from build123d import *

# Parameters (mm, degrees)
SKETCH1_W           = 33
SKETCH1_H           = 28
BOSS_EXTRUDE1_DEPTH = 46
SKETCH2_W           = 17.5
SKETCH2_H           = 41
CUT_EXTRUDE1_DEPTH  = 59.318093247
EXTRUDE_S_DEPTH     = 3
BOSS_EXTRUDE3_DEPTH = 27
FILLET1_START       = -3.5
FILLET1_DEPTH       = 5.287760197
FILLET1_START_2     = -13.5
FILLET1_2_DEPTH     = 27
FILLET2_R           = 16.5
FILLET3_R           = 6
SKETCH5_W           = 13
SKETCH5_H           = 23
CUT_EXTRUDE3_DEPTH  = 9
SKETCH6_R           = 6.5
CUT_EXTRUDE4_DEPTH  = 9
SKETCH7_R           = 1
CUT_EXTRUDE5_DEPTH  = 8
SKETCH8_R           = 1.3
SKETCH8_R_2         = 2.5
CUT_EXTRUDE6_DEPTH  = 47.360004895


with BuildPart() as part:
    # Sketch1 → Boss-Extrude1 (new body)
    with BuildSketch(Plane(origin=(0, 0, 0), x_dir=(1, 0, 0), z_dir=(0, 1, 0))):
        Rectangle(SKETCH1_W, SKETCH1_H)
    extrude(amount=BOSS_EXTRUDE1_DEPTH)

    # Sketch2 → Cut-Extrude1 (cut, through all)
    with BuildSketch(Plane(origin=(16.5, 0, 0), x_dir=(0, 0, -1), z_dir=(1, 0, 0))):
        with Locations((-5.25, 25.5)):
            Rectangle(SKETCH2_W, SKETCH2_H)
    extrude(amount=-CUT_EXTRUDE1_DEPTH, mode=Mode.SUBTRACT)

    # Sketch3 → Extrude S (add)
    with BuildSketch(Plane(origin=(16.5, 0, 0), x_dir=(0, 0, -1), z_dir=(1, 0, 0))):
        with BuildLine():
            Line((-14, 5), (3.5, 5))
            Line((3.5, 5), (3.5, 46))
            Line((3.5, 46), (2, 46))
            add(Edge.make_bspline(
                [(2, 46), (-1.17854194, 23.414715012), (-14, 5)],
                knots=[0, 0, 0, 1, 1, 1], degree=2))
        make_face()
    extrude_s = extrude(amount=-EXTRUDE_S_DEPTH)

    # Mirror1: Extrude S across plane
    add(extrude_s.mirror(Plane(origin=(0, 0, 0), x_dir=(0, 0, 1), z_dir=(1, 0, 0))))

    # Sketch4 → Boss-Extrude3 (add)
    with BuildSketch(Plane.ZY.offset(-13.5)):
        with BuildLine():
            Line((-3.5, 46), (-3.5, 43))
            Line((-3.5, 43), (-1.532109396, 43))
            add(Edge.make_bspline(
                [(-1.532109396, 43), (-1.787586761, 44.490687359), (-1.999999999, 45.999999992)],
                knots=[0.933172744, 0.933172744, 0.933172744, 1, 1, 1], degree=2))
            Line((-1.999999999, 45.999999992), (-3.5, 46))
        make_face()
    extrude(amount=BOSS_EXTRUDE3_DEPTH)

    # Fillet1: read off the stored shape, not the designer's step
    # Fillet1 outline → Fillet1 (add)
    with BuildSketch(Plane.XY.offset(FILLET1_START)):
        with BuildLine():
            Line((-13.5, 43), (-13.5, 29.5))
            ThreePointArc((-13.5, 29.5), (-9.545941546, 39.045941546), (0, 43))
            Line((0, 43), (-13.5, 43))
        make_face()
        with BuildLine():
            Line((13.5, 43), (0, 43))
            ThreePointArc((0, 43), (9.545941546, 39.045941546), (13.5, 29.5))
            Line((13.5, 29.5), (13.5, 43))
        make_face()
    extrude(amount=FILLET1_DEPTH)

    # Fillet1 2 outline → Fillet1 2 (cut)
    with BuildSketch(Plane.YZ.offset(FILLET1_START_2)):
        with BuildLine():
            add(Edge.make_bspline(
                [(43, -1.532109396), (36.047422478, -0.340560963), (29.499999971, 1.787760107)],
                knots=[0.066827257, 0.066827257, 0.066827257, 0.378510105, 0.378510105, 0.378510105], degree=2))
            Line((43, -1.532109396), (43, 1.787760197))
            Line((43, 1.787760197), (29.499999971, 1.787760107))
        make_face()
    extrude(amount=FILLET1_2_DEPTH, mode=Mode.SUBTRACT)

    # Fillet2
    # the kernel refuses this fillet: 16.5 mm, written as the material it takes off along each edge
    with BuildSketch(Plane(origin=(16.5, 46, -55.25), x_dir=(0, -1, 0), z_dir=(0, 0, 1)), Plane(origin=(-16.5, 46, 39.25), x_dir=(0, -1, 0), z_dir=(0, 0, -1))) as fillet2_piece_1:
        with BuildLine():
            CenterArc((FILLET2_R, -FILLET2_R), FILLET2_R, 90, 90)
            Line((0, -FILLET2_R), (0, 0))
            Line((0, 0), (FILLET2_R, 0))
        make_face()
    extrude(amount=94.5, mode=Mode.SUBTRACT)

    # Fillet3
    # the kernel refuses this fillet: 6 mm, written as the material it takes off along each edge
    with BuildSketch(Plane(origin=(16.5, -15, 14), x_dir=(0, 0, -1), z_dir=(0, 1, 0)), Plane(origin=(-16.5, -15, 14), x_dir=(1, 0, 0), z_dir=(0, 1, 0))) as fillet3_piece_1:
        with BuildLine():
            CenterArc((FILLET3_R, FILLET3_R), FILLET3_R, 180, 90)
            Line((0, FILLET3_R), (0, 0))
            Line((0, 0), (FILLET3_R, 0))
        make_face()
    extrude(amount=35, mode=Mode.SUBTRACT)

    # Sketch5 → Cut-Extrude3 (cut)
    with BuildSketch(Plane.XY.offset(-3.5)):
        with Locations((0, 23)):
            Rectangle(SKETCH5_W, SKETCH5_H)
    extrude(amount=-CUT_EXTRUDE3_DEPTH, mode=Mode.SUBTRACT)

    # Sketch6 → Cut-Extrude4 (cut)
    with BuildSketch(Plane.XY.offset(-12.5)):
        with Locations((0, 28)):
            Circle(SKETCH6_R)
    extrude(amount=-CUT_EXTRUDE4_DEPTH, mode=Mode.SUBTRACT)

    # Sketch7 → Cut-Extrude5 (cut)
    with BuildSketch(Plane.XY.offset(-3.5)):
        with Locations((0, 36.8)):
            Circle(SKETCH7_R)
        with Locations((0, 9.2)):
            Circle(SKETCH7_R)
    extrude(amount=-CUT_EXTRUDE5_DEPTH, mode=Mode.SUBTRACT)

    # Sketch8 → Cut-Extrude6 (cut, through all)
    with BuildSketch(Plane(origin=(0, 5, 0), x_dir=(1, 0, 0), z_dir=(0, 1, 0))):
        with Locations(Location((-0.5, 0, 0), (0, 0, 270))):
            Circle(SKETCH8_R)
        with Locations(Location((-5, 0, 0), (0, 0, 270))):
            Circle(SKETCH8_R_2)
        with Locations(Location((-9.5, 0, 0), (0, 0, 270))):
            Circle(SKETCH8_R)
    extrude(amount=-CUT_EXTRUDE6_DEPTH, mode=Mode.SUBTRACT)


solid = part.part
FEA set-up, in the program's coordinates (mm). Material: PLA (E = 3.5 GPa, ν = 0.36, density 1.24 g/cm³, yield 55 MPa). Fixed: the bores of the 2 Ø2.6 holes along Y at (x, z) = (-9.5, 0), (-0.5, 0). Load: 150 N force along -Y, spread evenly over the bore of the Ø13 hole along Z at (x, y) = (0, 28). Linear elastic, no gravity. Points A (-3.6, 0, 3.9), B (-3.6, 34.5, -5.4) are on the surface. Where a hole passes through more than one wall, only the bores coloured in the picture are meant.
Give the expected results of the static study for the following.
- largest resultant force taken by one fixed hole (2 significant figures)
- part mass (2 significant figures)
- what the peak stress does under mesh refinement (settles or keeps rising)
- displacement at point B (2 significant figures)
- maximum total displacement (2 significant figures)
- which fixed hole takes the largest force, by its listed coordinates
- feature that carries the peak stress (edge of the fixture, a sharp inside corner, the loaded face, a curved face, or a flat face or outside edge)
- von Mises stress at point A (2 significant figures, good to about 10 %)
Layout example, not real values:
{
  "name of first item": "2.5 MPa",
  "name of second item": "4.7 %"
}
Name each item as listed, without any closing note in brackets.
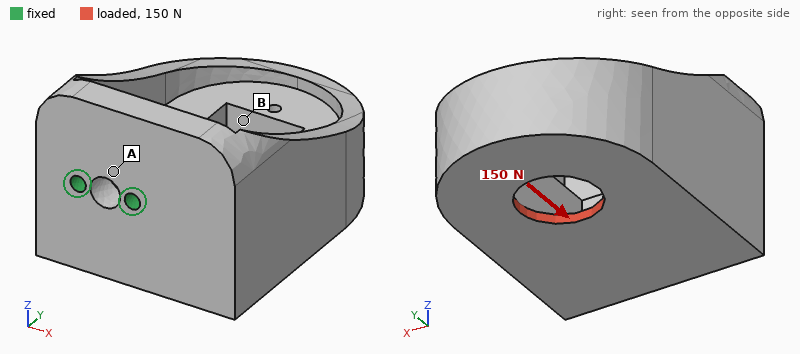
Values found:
{
  "largest resultant force taken by one fixed hole": "120 N",
  "part mass": "20 g",
  "what the peak stress does under mesh refinement": "keeps rising",
  "displacement at point B": "0.24 mm",
  "maximum total displacement": "0.36 mm",
  "which fixed hole takes the largest force, by its listed coordinates": "(-0.5, 0)",
  "feature that carries the peak stress": "edge of the fixture",
  "von Mises stress at point A": "4.2 MPa"
}
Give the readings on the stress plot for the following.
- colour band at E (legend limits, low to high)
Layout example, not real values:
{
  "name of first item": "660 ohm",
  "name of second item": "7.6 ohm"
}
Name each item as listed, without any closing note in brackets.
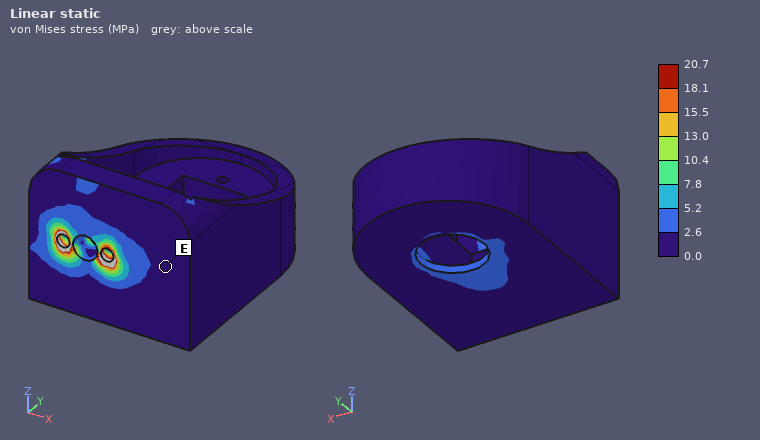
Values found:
{
  "colour band at E": "0.0 to 2.6 MPa"
}
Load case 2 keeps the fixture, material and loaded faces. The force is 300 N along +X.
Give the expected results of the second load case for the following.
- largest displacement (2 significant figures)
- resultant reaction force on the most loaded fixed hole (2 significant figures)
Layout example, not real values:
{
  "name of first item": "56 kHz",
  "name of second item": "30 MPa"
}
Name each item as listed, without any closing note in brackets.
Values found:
{
  "largest displacement": "0.65 mm",
  "resultant reaction force on the most loaded fixed hole": "640 N"
}
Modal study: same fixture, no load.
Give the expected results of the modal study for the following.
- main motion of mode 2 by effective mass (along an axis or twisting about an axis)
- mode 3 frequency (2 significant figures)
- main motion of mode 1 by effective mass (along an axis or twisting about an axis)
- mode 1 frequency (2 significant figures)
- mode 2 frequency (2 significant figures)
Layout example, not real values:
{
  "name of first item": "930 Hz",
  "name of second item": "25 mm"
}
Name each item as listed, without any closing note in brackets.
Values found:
{
  "main motion of mode 2 by effective mass": "along X",
  "mode 3 frequency": "2400 Hz",
  "main motion of mode 1 by effective mass": "along Z",
  "mode 1 frequency": "780 Hz",
  "mode 2 frequency": "1100 Hz"
}
